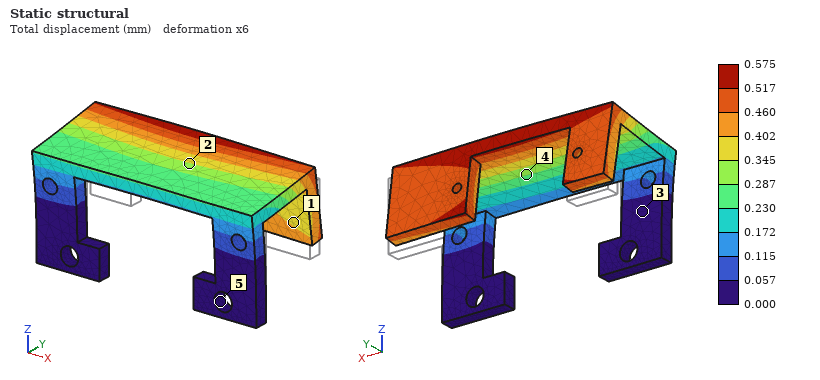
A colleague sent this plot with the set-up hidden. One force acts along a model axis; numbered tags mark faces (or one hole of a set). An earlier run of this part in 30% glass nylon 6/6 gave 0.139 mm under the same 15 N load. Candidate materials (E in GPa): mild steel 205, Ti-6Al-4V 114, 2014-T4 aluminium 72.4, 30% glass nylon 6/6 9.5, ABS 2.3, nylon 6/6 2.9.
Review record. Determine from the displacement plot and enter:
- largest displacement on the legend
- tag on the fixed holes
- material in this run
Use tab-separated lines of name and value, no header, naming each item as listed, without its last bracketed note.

largest displacement on the legend	0.575 mm
tag on the fixed holes	5
material in this run	ABS
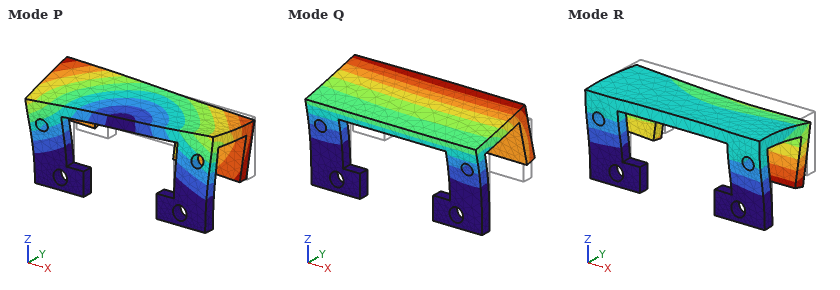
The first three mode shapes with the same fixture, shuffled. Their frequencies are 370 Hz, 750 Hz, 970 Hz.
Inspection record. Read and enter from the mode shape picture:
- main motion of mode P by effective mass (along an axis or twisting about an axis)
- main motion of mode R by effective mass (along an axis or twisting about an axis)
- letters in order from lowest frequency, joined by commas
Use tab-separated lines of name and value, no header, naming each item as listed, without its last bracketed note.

main motion of mode P by effective mass	along X
main motion of mode R by effective mass	along Y
letters in order from lowest frequency, joined by commas	Q, P, R
